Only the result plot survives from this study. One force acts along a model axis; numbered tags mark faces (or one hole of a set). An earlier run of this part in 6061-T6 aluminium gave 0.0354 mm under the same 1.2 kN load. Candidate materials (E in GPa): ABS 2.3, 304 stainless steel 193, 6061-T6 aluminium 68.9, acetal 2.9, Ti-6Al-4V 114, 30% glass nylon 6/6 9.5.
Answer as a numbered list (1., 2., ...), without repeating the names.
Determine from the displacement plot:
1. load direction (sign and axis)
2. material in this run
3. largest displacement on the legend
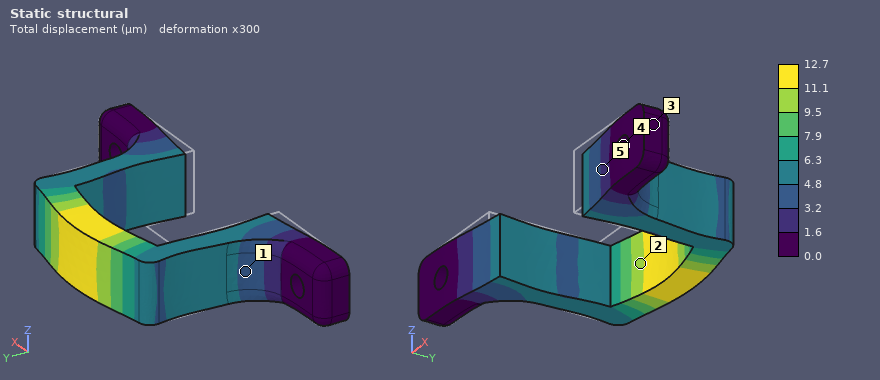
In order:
1. +Y
2. 304 stainless steel
3. 12.7 µm
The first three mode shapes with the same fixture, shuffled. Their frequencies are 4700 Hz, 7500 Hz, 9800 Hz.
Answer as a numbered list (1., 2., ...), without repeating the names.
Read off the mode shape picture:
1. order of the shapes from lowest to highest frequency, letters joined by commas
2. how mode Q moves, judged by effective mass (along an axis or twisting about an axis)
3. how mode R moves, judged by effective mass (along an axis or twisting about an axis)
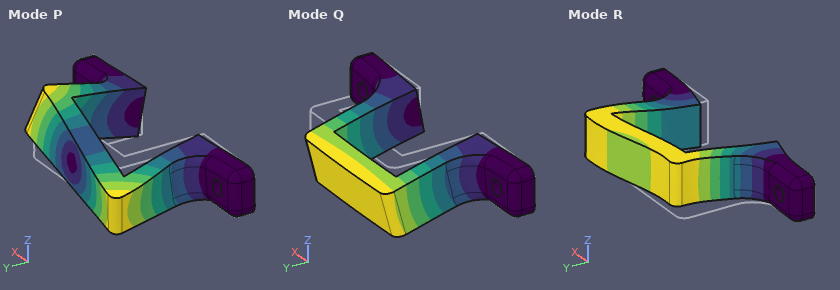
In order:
1. Q, R, P
2. along Z
3. along X
